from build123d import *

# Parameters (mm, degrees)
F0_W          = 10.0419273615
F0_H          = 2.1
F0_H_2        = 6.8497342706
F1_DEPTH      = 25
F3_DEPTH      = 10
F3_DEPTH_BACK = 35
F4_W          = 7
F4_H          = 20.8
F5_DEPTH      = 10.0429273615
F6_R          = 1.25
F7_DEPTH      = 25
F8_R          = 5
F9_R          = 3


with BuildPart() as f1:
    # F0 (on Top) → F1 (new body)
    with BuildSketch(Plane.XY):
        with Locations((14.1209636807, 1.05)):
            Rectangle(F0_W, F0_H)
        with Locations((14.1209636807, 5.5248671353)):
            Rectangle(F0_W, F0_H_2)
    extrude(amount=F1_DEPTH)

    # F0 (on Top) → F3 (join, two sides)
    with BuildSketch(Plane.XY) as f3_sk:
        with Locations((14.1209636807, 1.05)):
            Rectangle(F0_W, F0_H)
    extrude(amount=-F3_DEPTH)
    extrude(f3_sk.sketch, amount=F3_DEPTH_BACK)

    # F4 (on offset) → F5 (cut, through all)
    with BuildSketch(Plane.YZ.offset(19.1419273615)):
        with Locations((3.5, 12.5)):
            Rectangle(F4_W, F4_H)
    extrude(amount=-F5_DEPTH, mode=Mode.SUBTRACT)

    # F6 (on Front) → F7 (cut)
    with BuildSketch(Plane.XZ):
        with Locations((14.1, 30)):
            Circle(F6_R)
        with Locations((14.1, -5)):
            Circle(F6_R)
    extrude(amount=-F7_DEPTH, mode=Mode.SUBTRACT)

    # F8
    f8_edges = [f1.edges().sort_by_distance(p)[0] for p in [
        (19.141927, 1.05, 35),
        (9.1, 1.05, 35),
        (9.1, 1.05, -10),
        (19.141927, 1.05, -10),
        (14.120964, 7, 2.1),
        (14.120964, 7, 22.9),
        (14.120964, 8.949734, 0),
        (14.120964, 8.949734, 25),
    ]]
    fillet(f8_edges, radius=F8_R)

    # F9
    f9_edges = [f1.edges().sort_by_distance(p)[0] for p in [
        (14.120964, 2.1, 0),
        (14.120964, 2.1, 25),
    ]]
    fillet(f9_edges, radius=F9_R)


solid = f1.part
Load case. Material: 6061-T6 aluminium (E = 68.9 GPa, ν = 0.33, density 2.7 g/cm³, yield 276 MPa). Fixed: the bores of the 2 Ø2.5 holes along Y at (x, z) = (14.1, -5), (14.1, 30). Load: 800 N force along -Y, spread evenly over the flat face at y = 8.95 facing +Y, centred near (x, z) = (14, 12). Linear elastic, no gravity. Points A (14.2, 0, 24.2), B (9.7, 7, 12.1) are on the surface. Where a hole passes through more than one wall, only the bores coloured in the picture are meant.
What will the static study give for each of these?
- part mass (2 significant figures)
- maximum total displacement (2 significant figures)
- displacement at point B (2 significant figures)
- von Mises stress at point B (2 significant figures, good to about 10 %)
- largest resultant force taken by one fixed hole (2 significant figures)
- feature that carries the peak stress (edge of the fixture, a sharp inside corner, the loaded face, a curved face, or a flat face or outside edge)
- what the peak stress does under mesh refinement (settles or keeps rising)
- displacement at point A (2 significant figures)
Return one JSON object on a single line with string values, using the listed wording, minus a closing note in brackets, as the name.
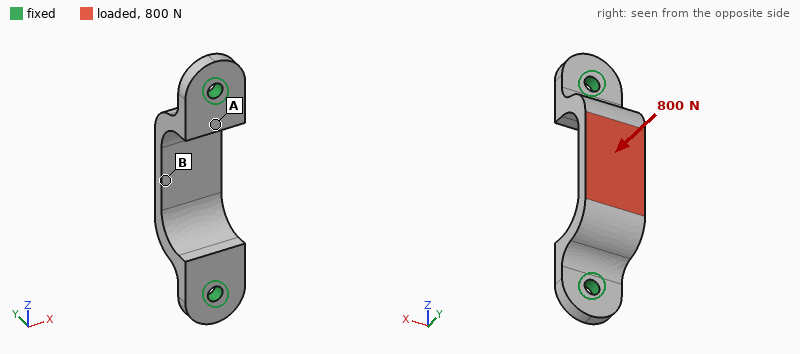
{"part mass": "3.2 g", "maximum total displacement": "52 µm", "displacement at point B": "51 µm", "von Mises stress at point B": "78 MPa", "largest resultant force taken by one fixed hole": "690 N", "feature that carries the peak stress": "edge of the fixture", "what the peak stress does under mesh refinement": "keeps rising", "displacement at point A": "10 µm"}
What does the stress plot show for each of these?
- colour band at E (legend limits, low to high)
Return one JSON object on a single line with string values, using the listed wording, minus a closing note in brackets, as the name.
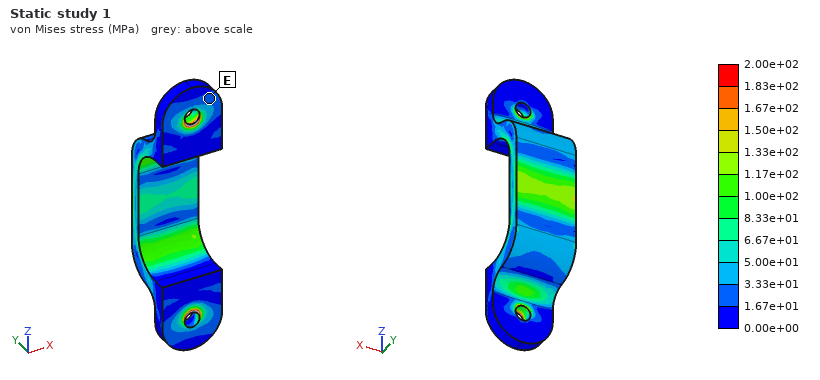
{"colour band at E": "1.67e+01 to 3.33e+01 MPa"}
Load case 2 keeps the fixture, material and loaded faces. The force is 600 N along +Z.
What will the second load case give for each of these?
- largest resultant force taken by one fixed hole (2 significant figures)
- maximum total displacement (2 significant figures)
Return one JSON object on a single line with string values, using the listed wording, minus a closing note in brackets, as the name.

{"largest resultant force taken by one fixed hole": "330 N", "maximum total displacement": "29 µm"}
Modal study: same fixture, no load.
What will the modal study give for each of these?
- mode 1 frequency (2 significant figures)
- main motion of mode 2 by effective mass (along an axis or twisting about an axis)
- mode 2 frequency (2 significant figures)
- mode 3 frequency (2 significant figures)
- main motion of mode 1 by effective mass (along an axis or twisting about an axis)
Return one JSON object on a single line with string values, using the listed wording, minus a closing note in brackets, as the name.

{"mode 1 frequency": "11 kHz", "main motion of mode 2 by effective mass": "along Z", "mode 2 frequency": "16 kHz", "mode 3 frequency": "21 kHz", "main motion of mode 1 by effective mass": "along X"}
